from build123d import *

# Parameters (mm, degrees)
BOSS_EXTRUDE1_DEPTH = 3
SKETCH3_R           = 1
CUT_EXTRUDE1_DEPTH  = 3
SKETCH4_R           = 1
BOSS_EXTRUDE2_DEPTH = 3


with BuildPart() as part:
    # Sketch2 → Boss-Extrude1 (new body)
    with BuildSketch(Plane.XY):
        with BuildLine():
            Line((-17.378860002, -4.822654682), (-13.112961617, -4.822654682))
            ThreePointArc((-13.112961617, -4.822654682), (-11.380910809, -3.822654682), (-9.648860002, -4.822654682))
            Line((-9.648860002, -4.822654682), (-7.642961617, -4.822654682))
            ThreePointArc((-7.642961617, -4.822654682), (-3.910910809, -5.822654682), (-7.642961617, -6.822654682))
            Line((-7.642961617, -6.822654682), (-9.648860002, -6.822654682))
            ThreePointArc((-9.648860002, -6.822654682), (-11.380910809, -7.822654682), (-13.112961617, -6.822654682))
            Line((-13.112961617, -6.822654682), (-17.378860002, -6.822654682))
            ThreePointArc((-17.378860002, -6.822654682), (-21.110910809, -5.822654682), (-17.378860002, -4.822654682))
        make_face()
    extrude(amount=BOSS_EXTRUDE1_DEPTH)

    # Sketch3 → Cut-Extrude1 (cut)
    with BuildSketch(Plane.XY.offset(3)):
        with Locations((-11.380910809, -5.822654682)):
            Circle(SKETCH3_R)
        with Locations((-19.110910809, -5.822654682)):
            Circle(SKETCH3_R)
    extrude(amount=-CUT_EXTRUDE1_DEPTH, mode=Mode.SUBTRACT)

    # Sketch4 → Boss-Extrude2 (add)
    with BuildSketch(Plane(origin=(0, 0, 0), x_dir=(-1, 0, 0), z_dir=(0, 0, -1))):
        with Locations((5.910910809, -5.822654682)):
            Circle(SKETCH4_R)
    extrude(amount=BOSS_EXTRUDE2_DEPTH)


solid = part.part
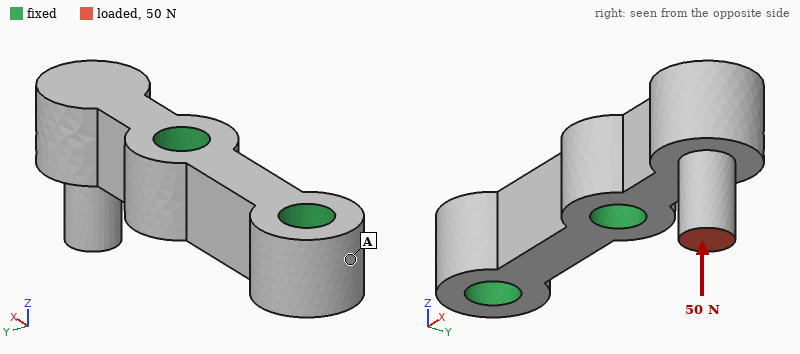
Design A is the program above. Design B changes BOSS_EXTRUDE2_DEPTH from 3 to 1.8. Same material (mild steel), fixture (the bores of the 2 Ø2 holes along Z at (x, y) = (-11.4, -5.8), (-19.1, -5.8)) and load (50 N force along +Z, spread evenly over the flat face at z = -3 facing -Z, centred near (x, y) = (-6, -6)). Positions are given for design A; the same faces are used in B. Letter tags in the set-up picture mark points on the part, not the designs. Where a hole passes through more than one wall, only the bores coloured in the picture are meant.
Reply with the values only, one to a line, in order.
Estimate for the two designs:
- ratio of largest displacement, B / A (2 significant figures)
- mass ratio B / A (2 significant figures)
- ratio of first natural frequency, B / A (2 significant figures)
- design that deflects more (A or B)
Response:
0.88
0.97
1.1
A
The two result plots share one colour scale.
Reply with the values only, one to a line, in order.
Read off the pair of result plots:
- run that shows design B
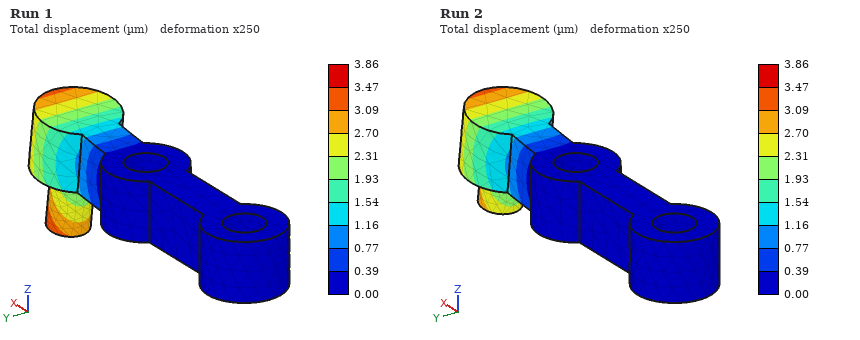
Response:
Run 2
